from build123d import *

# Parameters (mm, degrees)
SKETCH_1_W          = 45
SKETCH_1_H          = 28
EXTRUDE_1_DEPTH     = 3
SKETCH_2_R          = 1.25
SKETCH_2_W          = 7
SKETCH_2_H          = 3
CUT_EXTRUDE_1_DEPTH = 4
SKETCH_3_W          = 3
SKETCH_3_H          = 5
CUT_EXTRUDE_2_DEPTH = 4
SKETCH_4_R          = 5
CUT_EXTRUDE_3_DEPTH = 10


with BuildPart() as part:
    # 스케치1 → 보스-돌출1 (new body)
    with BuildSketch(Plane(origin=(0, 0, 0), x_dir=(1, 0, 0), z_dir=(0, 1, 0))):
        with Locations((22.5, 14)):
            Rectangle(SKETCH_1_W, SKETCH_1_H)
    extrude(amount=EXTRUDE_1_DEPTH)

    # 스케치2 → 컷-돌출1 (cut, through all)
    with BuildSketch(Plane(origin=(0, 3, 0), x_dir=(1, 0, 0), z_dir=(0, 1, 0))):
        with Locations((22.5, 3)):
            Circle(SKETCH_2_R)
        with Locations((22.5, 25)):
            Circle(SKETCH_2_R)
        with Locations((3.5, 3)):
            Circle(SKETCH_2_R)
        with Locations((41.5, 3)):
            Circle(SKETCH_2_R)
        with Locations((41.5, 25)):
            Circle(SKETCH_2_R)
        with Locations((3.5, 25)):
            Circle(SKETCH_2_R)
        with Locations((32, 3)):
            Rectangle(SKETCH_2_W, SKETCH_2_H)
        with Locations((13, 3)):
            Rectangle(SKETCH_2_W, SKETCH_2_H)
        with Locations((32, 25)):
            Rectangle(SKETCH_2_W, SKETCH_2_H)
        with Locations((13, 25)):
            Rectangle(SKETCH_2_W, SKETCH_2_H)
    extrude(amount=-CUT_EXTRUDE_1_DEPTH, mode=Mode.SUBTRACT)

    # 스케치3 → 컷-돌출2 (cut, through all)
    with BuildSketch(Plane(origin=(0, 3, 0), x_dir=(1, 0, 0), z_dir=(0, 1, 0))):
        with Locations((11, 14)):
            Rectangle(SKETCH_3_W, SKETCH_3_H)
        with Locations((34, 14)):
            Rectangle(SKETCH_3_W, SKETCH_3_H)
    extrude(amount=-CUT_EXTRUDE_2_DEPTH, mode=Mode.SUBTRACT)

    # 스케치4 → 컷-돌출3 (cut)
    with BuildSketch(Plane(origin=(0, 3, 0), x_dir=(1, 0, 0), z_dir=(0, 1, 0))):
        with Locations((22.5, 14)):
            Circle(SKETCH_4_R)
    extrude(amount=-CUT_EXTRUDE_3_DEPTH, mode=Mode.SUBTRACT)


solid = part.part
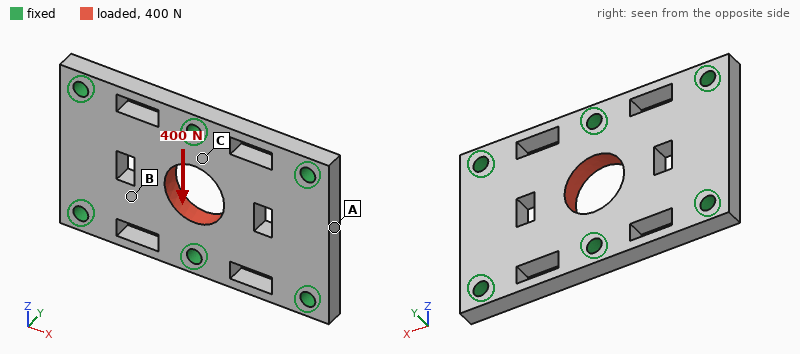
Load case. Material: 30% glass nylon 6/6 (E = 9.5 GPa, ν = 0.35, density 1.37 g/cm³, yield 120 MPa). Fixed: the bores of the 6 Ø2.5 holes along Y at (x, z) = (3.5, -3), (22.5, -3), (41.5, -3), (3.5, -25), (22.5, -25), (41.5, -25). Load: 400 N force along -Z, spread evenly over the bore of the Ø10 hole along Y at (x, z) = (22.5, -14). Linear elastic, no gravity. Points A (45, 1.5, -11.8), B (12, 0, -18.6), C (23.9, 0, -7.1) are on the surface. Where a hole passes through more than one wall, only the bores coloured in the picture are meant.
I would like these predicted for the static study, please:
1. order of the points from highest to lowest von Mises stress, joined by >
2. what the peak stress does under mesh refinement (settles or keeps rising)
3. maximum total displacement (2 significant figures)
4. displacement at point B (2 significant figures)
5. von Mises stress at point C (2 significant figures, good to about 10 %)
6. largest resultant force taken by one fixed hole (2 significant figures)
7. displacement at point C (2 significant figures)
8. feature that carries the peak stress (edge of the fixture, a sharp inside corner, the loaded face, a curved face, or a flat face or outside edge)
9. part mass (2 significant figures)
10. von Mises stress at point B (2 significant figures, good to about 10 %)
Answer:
C > B > A
keeps rising
6.2 µm
2.6 µm
6.8 MPa
160 N
2.9 µm
edge of the fixture
4.3 g
2.3 MPa
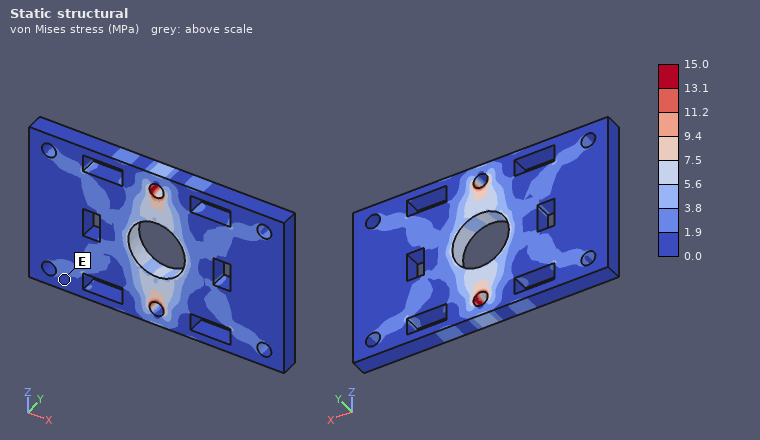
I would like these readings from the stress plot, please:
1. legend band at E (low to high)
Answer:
0.0 to 1.9 MPa
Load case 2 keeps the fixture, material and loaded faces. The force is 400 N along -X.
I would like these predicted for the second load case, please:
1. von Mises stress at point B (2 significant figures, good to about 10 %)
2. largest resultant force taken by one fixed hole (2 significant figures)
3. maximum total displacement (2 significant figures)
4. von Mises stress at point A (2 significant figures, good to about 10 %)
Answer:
3.4 MPa
100 N
7.4 µm
1.3 MPa
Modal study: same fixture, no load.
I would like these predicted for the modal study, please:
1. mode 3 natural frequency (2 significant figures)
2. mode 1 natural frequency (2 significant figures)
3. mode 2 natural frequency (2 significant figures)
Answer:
19 kHz
13 kHz
13 kHz
